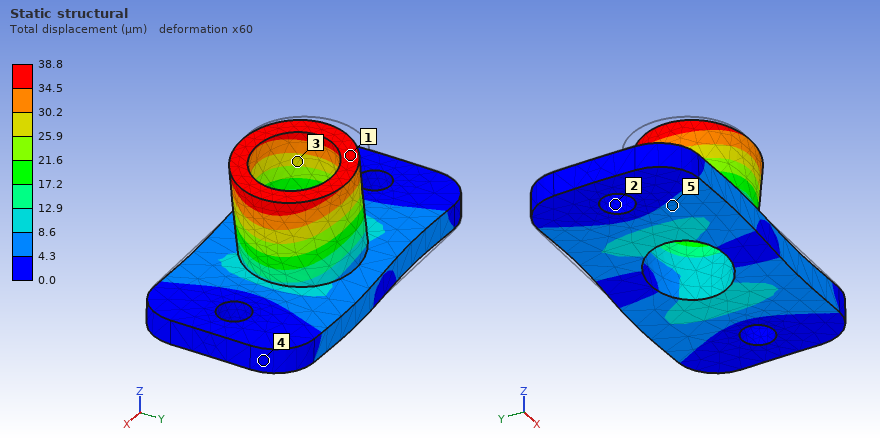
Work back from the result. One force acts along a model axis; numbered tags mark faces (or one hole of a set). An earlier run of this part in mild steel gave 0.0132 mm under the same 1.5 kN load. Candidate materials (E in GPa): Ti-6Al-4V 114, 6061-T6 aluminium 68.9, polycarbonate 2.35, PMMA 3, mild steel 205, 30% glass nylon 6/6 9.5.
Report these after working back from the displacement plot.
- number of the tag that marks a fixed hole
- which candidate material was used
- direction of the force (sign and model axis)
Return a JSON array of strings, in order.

["2", "6061-T6 aluminium", "+X"]
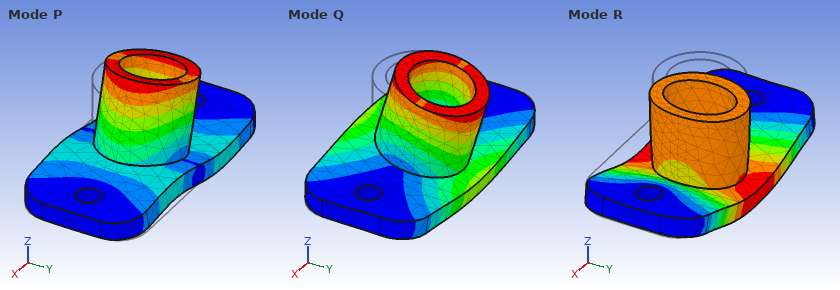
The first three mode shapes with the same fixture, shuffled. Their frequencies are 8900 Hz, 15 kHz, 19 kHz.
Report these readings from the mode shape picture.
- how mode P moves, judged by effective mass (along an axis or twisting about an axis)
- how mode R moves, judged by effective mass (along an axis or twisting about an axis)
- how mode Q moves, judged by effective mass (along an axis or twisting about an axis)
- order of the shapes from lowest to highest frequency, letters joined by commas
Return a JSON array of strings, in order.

["along X", "along Z", "along Y", "Q, R, P"]
